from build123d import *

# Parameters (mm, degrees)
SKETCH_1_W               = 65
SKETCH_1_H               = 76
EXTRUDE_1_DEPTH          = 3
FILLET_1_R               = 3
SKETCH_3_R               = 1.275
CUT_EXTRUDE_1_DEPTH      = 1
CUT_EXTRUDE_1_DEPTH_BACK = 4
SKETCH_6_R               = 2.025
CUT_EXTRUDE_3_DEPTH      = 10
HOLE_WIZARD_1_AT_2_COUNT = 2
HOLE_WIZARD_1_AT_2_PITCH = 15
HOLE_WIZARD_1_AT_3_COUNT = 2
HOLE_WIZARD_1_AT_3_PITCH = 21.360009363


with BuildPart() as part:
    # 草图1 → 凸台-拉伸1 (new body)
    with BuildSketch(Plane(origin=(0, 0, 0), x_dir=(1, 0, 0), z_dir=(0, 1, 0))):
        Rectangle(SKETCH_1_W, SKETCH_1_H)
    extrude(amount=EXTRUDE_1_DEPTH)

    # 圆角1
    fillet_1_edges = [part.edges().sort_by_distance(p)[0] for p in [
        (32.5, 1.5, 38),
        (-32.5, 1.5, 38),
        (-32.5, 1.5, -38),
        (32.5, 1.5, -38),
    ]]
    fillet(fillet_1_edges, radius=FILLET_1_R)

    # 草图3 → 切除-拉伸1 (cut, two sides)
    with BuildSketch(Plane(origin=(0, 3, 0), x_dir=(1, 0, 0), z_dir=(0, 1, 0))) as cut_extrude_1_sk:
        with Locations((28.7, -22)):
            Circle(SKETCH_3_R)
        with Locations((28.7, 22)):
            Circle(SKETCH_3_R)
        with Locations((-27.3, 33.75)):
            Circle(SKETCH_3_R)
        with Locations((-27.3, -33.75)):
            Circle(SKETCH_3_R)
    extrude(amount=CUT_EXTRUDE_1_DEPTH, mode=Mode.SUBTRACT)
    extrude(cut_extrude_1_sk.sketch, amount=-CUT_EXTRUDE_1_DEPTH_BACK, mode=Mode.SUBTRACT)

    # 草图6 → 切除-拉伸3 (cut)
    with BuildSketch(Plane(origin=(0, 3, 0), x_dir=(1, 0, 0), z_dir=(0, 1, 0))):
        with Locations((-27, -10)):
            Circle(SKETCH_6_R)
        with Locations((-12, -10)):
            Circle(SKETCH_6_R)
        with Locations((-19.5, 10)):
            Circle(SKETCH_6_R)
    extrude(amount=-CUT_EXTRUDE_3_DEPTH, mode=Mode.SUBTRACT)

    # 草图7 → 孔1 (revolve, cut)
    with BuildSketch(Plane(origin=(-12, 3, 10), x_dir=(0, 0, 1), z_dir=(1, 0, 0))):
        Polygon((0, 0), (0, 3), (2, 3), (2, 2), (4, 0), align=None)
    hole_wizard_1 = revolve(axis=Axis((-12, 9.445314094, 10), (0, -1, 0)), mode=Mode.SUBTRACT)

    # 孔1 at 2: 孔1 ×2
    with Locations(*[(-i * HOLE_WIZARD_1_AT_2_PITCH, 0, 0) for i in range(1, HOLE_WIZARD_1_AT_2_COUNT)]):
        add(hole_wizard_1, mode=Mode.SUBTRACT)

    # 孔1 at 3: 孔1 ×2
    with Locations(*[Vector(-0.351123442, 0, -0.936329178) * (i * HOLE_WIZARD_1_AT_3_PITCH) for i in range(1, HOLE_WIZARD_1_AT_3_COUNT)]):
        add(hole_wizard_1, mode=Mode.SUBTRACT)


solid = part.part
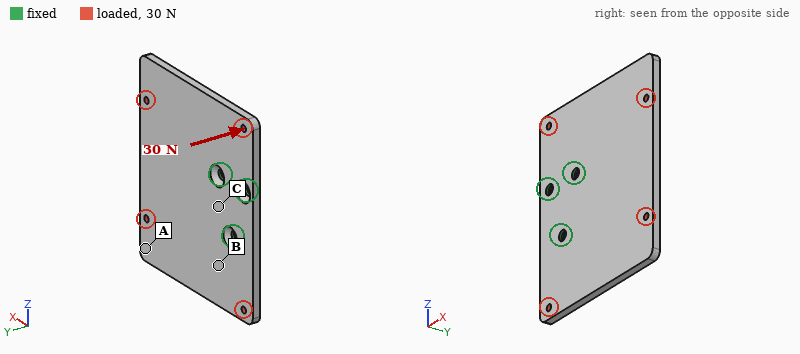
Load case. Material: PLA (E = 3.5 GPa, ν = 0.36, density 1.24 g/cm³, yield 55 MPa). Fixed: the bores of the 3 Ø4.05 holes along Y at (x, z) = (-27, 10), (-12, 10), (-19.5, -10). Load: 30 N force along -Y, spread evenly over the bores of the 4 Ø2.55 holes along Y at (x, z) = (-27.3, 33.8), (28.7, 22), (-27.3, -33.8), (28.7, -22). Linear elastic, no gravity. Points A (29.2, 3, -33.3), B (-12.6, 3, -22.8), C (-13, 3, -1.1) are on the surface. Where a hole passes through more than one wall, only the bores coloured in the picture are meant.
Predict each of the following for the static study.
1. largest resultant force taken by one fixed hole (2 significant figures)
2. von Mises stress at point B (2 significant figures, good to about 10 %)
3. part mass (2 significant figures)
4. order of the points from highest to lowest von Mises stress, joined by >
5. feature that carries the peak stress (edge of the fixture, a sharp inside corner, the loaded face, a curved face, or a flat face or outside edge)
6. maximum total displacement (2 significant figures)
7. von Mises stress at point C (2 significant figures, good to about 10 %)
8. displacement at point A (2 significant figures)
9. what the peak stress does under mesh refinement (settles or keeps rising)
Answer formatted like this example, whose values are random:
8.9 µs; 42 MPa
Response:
43 N; 3.2 MPa; 18 g; C > B > A; edge of the fixture; 1.2 mm; 5.7 MPa; 1.1 mm; keeps rising
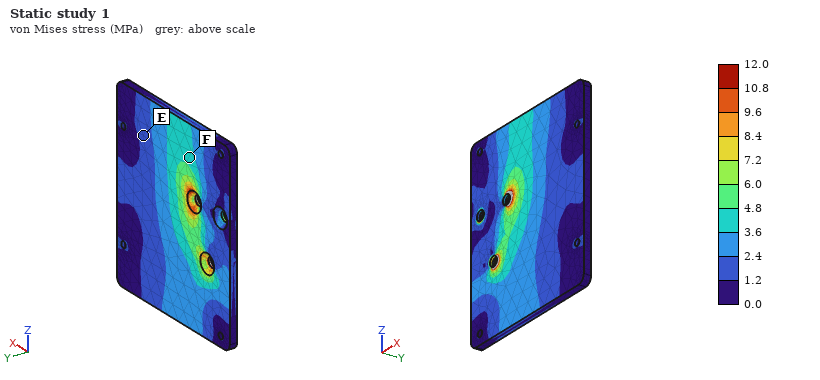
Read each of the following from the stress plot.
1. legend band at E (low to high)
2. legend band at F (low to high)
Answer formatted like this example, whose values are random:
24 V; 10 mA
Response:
1.2 to 2.4 MPa; 3.6 to 4.8 MPa
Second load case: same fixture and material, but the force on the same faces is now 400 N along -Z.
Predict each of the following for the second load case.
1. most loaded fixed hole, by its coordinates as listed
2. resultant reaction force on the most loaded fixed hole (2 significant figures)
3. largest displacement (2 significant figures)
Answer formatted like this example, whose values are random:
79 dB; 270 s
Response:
(-12, 10); 350 N; 0.20 mm
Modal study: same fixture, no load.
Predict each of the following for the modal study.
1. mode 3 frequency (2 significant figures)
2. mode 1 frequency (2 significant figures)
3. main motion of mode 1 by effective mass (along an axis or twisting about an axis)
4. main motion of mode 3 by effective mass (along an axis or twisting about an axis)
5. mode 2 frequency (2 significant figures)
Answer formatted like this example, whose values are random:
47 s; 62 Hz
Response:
850 Hz; 290 Hz; along Y; along Y; 440 Hz
